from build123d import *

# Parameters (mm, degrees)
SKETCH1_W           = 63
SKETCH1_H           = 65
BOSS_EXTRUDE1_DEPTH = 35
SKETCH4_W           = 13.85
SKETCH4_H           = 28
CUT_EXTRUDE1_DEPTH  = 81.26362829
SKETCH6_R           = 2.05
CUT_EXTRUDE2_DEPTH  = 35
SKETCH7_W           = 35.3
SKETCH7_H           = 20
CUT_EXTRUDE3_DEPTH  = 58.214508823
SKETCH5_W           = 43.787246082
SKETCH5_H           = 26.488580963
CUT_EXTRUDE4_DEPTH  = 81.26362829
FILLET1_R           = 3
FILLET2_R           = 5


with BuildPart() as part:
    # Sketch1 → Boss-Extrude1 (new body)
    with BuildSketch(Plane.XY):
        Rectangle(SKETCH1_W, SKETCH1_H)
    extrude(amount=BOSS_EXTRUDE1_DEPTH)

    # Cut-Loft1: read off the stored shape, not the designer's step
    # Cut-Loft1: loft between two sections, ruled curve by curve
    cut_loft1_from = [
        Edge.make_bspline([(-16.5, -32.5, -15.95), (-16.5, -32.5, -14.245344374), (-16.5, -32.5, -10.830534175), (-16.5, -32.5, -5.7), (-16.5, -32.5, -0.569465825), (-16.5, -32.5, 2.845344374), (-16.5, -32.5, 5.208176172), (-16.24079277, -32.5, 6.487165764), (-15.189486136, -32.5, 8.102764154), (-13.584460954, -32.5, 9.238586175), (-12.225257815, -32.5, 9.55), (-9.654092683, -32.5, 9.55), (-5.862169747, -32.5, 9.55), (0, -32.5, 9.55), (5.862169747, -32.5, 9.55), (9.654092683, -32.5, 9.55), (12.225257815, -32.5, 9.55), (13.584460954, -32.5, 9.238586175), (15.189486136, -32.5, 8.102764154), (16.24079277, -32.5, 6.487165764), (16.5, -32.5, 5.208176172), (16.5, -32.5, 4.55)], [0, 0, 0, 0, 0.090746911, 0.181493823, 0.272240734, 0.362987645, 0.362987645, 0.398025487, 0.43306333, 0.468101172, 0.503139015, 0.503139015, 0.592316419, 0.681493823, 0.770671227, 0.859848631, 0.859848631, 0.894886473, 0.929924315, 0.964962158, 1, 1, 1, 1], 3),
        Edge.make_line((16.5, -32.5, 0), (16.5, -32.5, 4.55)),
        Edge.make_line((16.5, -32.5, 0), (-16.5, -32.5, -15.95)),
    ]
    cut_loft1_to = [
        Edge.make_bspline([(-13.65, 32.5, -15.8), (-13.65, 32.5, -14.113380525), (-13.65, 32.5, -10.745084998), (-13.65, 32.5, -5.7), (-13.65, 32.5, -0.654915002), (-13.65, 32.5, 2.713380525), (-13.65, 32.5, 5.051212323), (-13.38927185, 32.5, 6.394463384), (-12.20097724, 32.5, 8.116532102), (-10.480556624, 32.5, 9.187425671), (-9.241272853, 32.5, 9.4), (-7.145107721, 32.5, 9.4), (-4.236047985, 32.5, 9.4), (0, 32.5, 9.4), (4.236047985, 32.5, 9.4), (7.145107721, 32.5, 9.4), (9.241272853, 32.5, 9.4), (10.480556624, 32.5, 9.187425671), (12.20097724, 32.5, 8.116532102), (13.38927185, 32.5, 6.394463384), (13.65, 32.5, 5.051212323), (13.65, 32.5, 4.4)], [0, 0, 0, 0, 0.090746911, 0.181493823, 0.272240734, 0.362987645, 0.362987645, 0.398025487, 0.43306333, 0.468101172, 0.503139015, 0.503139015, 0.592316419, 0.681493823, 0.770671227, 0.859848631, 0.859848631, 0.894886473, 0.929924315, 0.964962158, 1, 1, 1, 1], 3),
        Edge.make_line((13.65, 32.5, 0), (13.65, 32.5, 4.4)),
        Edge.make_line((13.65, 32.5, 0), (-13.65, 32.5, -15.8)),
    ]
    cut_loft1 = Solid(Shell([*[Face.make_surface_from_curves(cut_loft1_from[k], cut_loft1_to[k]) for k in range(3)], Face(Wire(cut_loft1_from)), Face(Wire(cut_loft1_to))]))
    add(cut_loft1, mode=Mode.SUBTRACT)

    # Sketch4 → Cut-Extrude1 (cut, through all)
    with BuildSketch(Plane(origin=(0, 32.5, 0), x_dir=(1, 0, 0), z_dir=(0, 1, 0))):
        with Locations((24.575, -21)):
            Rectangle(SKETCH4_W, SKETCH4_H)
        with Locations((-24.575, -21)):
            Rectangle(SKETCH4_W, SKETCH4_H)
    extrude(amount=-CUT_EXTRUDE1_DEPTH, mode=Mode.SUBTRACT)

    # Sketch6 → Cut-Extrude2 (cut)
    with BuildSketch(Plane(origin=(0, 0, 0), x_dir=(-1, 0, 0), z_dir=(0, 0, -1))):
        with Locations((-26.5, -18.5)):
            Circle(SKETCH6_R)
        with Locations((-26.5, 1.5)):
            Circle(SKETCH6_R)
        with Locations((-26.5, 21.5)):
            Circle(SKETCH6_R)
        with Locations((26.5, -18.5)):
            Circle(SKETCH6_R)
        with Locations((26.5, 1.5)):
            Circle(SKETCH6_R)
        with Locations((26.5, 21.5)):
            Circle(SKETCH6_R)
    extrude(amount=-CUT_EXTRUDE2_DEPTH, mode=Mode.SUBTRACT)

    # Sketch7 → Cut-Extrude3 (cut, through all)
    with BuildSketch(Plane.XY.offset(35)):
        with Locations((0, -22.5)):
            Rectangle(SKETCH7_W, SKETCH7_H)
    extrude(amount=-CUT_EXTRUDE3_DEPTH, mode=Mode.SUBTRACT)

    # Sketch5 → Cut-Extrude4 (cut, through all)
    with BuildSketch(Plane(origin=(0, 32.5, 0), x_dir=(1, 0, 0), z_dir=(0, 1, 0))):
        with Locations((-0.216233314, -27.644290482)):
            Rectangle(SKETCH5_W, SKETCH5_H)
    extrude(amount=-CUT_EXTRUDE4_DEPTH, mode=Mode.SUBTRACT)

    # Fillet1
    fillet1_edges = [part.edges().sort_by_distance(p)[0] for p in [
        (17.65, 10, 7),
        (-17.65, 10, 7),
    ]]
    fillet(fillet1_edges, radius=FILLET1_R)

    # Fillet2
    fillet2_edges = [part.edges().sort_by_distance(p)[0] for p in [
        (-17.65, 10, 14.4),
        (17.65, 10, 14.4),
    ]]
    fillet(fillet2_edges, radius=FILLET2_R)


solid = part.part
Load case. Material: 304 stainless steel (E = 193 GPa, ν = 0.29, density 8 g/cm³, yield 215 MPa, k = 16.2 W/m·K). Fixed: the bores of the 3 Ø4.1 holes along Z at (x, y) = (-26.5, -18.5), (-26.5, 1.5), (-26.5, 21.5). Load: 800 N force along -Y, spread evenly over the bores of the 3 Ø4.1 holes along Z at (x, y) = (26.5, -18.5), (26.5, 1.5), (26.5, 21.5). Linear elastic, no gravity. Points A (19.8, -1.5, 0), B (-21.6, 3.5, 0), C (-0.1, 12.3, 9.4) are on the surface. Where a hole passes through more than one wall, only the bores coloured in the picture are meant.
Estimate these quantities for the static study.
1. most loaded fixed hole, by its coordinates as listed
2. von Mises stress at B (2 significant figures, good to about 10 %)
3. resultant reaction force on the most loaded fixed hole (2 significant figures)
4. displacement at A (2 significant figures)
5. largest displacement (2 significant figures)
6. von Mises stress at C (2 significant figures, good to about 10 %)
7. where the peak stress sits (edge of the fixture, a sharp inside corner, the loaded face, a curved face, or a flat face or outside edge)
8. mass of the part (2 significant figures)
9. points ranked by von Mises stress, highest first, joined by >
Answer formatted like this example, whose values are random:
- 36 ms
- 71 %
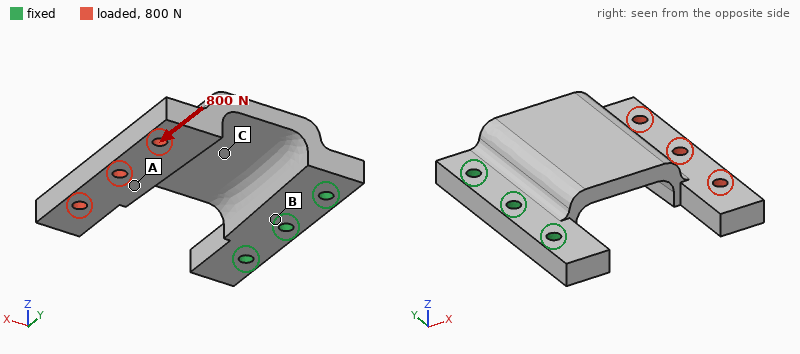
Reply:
- (-26.5, 21.5)
- 24 MPa
- 1.4 kN
- 46 µm
- 89 µm
- 38 MPa
- a curved face
- 180 g
- C > B > A
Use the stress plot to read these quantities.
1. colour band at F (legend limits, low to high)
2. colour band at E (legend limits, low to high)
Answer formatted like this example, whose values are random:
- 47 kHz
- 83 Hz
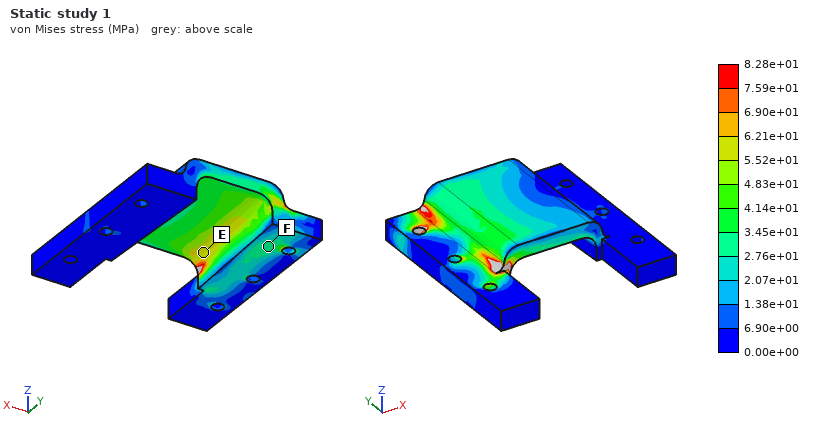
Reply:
- 2.76e+01 to 3.45e+01 MPa
- 5.52e+01 to 6.21e+01 MPa
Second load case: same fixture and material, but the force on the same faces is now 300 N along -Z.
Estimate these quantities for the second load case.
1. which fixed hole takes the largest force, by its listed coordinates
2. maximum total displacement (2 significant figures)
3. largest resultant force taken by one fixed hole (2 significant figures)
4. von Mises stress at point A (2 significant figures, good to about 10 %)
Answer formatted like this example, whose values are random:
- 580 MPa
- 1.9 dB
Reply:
- (-26.5, 1.5)
- 0.20 mm
- 220 N
- 9.5 MPa
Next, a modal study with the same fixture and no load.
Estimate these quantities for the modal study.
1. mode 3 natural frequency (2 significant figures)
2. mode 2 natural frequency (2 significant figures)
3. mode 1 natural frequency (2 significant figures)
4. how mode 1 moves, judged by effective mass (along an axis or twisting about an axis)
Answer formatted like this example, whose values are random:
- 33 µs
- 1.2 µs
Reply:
- 3500 Hz
- 2000 Hz
- 920 Hz
- along Z
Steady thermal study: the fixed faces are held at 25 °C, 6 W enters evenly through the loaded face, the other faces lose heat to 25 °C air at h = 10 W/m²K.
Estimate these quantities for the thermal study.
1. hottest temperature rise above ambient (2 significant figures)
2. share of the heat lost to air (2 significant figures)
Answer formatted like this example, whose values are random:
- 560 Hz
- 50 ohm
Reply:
- 69 K
- 46 %
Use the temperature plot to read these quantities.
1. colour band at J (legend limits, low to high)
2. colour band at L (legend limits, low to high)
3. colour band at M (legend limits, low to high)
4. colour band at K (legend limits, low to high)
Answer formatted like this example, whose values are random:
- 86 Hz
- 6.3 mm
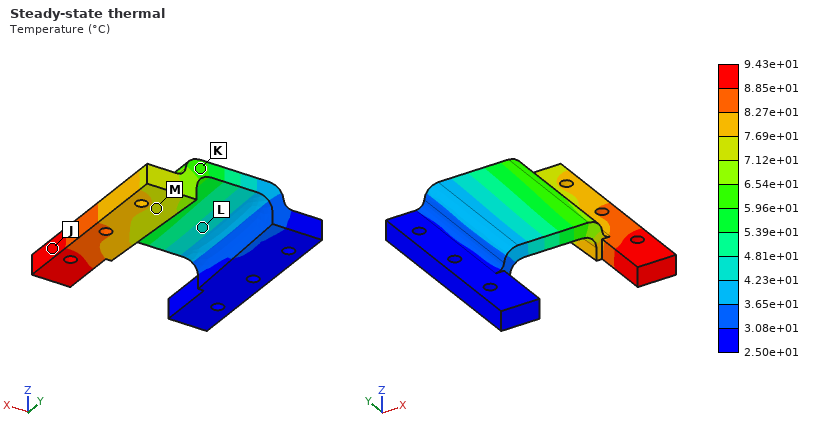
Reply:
- 8.85e+01 to 9.43e+01 °C
- 4.23e+01 to 4.81e+01 °C
- 7.12e+01 to 7.69e+01 °C
- 5.96e+01 to 6.54e+01 °C
